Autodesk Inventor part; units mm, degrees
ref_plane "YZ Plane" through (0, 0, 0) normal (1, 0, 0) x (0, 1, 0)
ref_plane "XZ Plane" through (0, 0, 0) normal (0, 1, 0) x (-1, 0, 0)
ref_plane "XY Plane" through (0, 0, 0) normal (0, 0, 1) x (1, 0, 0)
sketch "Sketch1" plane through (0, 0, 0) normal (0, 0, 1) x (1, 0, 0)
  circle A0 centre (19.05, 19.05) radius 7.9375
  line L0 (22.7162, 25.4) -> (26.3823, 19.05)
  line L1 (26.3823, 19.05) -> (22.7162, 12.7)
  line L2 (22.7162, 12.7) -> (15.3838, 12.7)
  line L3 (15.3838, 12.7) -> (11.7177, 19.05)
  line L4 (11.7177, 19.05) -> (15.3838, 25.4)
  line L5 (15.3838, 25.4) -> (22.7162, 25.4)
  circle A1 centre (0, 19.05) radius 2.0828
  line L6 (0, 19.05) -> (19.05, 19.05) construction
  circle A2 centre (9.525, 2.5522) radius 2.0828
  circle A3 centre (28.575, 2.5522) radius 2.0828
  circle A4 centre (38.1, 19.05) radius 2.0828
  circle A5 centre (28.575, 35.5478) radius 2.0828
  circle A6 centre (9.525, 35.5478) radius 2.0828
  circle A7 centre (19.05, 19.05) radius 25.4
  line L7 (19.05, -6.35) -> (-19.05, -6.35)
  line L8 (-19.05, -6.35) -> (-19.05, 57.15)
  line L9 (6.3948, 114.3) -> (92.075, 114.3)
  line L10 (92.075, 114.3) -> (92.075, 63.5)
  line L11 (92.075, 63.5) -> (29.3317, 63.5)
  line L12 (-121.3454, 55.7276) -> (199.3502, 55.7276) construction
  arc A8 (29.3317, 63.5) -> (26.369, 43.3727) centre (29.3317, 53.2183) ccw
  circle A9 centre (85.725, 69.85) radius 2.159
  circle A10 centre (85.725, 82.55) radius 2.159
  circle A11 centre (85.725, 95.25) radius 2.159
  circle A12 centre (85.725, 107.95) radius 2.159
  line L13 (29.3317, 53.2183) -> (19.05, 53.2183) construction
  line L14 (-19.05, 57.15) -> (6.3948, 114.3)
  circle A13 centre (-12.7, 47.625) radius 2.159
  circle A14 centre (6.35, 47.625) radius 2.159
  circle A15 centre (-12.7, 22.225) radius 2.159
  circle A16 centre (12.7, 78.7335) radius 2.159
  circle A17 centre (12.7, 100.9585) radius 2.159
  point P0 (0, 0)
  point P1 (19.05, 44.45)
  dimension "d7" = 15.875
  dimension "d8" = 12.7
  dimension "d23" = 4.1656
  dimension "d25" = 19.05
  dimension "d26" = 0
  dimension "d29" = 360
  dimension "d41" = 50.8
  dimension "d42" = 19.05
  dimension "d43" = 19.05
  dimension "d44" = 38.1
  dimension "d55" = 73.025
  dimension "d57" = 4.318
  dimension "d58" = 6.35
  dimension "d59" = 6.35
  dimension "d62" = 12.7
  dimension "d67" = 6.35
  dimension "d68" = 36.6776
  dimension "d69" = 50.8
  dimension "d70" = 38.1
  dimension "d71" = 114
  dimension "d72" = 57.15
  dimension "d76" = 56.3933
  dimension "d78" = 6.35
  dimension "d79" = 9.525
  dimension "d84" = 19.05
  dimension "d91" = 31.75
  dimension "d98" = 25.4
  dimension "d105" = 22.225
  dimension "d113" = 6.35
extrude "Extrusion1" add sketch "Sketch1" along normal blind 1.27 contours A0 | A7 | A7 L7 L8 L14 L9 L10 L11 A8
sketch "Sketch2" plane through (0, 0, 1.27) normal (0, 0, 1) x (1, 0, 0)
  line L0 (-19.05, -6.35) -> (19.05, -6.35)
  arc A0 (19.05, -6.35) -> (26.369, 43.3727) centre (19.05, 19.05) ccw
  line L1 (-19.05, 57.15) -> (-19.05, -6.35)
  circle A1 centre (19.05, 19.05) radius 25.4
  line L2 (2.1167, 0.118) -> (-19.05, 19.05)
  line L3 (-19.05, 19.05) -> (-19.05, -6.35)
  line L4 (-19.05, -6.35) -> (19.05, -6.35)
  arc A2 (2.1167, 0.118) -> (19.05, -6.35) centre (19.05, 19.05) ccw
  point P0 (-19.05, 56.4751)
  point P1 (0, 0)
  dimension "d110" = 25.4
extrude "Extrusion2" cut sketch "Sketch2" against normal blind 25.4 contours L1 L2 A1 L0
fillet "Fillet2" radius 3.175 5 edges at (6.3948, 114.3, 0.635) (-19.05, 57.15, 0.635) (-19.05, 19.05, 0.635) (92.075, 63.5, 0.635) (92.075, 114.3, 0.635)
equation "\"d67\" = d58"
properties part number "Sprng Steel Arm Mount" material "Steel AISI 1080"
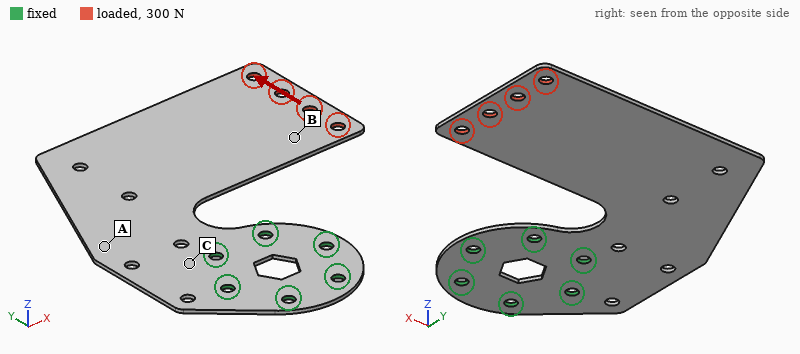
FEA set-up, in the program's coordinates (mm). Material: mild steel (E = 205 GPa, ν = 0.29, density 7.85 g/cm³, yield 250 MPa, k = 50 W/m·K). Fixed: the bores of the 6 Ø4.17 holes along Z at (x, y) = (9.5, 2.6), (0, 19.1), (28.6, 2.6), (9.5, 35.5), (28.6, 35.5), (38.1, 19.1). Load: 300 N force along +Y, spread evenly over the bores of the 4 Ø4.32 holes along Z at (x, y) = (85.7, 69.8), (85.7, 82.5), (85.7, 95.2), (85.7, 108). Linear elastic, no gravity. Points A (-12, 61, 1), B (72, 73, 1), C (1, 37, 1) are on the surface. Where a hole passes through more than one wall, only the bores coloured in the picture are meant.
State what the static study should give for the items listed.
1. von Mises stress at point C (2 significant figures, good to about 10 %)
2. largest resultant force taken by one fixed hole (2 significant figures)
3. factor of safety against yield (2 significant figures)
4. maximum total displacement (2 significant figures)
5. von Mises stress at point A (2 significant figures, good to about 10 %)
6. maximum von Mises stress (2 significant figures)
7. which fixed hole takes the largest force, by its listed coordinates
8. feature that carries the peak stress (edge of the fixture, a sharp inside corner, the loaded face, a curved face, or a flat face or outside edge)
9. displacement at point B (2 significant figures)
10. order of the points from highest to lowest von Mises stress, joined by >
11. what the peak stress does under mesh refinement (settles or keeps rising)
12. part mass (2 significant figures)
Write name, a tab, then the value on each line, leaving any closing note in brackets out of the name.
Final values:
von Mises stress at point C	27 MPa
largest resultant force taken by one fixed hole	560 N
factor of safety against yield	1.4
maximum total displacement	0.15 mm
von Mises stress at point A	49 MPa
maximum von Mises stress	170 MPa
which fixed hole takes the largest force, by its listed coordinates	(0, 19.1)
feature that carries the peak stress	a curved face
displacement at point B	0.097 mm
order of the points from highest to lowest von Mises stress, joined by >	A > C > B
what the peak stress does under mesh refinement	settles
part mass	79 g
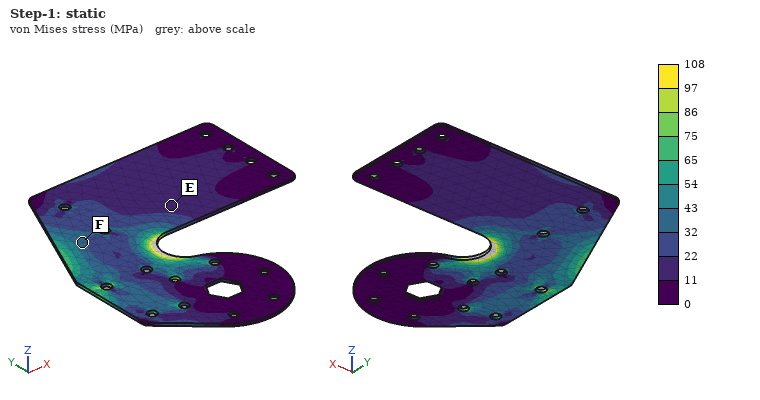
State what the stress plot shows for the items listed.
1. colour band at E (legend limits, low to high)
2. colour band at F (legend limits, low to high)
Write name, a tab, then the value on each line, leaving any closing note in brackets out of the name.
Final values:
colour band at E	11 to 22 MPa
colour band at F	32 to 43 MPa
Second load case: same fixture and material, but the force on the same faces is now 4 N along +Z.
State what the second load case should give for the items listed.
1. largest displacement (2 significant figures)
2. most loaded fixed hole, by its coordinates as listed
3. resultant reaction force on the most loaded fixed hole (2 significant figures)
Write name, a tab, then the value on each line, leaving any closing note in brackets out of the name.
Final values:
largest displacement	1.1 mm
most loaded fixed hole, by its coordinates as listed	(28.6, 35.5)
resultant reaction force on the most loaded fixed hole	8.2 N
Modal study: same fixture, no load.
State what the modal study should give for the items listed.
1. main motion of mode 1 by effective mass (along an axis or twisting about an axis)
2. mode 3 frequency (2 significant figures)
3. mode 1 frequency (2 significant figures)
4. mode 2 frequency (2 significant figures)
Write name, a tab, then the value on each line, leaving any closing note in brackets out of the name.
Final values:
main motion of mode 1 by effective mass	along Z
mode 3 frequency	540 Hz
mode 1 frequency	77 Hz
mode 2 frequency	190 Hz
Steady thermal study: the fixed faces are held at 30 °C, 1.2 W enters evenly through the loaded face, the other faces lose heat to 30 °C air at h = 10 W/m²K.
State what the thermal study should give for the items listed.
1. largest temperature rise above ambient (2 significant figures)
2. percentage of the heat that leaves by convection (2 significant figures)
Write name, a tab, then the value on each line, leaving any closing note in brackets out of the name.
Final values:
largest temperature rise above ambient	19 K
percentage of the heat that leaves by convection	84 %
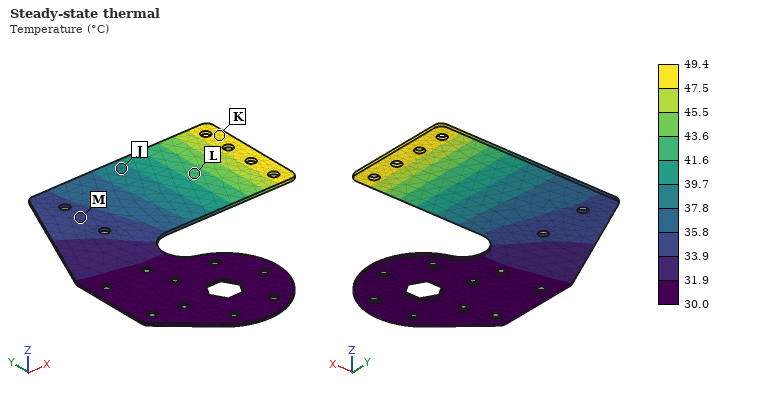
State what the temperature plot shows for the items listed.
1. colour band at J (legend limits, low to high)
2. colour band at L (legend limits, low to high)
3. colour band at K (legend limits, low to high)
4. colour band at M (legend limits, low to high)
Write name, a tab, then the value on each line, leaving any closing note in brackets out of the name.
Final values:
colour band at J	37.8 to 39.7 °C
colour band at L	41.6 to 43.6 °C
colour band at K	47.5 to 49.4 °C
colour band at M	33.9 to 35.8 °C
